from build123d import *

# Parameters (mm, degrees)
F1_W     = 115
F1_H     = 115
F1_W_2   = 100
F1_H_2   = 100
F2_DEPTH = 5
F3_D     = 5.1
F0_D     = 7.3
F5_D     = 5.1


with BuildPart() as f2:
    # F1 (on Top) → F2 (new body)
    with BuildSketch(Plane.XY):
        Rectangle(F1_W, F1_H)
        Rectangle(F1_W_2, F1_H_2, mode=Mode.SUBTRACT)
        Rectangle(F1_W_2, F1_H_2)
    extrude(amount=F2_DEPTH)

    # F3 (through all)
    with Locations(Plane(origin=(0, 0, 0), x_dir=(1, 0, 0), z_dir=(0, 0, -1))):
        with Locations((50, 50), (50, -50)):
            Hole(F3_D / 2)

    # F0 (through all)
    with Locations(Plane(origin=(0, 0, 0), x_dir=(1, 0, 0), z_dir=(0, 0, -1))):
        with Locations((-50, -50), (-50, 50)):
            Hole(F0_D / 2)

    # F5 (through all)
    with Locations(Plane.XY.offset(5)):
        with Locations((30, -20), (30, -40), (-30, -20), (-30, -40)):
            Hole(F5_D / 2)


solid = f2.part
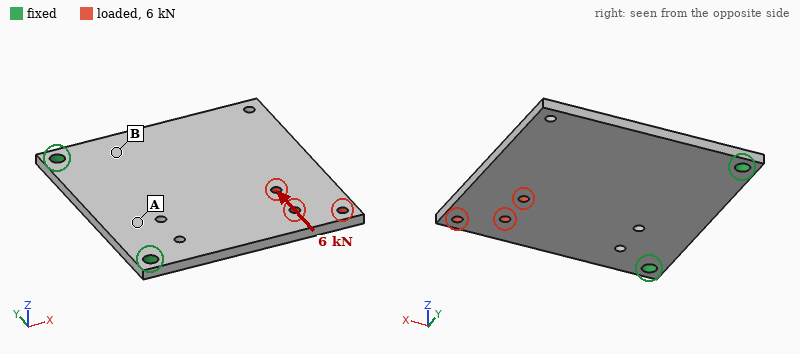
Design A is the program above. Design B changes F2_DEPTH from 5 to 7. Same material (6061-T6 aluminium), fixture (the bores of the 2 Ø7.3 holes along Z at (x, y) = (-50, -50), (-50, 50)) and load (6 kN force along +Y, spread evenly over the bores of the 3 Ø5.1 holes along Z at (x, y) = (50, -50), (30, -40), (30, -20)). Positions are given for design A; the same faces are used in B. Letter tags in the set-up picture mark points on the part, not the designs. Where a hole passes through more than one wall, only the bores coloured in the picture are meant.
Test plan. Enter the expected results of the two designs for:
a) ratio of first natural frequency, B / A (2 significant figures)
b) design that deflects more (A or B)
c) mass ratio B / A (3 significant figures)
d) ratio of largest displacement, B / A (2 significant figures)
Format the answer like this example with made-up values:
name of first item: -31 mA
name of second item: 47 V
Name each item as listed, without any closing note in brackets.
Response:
ratio of first natural frequency, B / A: 1.4
design that deflects more: A
mass ratio B / A: 1.40
ratio of largest displacement, B / A: 0.71
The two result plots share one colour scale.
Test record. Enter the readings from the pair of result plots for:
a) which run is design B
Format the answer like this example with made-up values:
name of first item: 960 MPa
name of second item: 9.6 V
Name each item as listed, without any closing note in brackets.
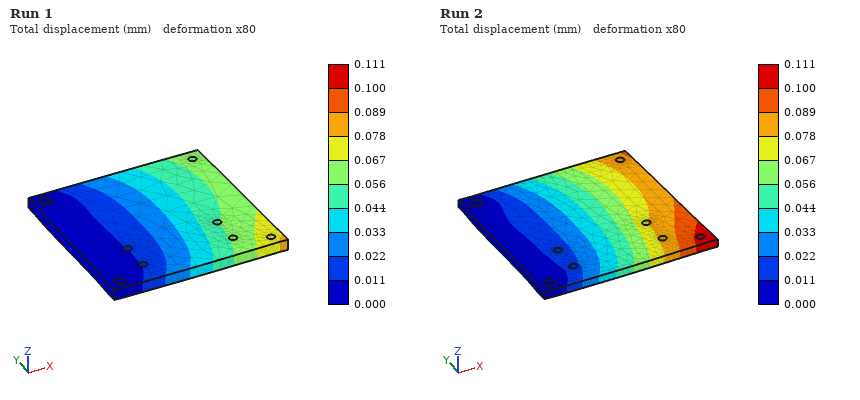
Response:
which run is design B: Run 1
